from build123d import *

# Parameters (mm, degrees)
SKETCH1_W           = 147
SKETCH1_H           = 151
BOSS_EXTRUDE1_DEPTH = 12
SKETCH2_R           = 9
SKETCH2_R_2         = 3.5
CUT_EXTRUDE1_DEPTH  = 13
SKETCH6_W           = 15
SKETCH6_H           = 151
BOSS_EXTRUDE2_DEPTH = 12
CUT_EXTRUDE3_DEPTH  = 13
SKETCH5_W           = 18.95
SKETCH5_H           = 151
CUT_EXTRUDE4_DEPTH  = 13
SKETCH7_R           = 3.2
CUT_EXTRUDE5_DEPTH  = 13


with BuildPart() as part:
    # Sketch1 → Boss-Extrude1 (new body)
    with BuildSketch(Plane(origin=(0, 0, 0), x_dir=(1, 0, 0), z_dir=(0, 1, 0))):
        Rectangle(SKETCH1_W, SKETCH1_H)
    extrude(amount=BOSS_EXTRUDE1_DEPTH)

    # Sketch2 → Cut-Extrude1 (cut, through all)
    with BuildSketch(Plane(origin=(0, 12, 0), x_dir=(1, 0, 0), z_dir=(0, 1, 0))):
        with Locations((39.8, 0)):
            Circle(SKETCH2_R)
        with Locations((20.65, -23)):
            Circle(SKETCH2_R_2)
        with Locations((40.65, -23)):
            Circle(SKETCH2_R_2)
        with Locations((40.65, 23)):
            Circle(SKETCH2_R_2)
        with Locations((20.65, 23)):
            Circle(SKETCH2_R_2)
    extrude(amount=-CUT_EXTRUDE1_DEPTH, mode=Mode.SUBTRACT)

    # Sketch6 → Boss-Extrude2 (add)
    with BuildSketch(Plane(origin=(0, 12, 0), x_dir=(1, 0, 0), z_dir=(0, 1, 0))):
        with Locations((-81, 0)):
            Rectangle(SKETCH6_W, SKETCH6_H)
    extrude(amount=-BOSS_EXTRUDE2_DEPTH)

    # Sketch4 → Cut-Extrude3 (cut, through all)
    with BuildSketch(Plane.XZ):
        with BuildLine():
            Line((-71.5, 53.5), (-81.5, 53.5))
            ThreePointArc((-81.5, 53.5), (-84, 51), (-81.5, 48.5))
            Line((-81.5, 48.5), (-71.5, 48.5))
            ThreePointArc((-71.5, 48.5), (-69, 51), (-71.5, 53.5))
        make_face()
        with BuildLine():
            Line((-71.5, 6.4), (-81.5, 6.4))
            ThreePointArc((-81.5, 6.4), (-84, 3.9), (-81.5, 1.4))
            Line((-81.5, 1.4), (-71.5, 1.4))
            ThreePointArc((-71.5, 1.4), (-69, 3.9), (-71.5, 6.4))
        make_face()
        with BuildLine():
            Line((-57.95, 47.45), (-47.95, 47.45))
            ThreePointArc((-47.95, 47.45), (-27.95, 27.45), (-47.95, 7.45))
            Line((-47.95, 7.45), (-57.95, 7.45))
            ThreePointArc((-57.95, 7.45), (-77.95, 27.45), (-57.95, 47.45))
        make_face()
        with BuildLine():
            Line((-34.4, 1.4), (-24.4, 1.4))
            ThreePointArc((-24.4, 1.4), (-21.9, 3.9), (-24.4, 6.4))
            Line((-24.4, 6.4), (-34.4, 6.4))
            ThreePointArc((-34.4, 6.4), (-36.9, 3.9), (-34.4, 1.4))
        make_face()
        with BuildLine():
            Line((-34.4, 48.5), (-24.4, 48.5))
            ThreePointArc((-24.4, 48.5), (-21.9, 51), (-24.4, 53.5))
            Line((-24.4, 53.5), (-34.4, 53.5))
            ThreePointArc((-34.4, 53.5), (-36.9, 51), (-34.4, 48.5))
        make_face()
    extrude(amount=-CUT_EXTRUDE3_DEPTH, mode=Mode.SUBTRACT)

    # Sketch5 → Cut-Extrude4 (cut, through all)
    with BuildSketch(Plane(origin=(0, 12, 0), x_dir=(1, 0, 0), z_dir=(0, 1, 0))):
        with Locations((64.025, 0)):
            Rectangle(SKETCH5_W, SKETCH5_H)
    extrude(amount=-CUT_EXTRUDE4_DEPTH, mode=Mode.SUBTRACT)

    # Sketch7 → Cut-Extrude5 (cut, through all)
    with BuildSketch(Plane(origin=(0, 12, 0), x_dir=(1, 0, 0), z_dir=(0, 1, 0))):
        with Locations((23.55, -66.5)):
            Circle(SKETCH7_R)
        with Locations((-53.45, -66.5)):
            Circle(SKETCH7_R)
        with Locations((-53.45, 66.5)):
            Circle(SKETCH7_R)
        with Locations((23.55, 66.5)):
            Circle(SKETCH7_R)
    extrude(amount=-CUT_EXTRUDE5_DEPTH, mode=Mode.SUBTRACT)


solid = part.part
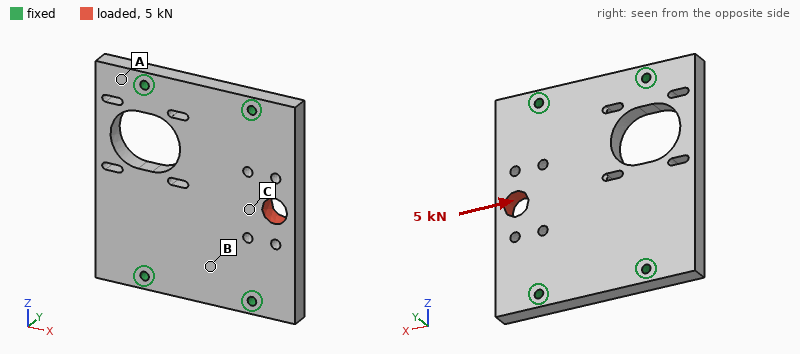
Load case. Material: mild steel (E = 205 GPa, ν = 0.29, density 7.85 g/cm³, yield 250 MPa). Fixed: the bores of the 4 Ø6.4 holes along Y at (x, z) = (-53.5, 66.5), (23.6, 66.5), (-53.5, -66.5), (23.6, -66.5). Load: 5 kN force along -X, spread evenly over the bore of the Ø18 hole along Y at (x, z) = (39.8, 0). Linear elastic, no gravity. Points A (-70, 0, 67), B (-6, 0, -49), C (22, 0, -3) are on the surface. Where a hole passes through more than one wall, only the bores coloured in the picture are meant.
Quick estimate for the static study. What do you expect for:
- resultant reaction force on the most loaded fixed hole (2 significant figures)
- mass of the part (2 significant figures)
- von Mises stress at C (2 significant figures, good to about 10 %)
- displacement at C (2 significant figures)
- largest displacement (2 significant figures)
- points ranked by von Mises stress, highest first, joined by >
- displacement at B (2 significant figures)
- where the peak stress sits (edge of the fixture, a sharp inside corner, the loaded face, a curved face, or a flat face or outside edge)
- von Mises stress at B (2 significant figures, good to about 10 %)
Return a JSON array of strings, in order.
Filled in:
["1.7 kN", "1.8 kg", "7.2 MPa", "3.0 µm", "5.2 µm", "C > B > A", "0.88 µm", "a flat face or outside edge", "4.4 MPa"]
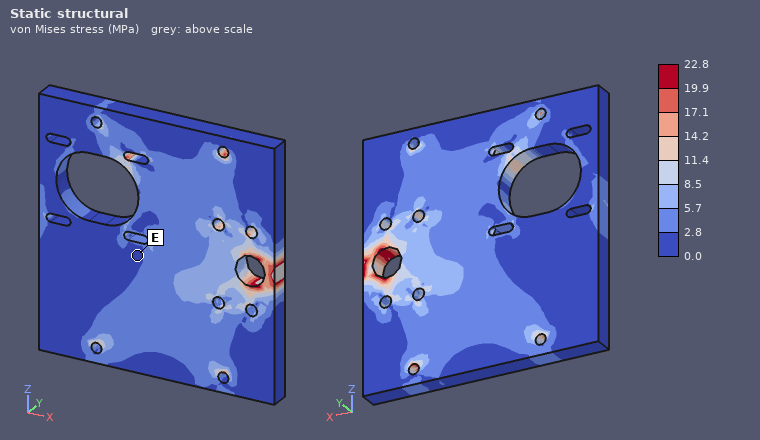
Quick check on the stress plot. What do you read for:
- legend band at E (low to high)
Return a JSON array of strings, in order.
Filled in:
["0.0 to 2.8 MPa"]
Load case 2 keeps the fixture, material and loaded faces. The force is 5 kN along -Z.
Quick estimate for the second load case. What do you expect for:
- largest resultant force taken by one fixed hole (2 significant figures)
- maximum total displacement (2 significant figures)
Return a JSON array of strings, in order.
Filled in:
["2.2 kN", "2.7 µm"]
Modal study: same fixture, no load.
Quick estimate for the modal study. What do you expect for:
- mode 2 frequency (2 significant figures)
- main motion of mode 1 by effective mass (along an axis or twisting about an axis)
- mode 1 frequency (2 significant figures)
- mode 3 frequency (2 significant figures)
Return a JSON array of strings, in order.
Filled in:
["3000 Hz", "along Y", "2500 Hz", "4400 Hz"]
